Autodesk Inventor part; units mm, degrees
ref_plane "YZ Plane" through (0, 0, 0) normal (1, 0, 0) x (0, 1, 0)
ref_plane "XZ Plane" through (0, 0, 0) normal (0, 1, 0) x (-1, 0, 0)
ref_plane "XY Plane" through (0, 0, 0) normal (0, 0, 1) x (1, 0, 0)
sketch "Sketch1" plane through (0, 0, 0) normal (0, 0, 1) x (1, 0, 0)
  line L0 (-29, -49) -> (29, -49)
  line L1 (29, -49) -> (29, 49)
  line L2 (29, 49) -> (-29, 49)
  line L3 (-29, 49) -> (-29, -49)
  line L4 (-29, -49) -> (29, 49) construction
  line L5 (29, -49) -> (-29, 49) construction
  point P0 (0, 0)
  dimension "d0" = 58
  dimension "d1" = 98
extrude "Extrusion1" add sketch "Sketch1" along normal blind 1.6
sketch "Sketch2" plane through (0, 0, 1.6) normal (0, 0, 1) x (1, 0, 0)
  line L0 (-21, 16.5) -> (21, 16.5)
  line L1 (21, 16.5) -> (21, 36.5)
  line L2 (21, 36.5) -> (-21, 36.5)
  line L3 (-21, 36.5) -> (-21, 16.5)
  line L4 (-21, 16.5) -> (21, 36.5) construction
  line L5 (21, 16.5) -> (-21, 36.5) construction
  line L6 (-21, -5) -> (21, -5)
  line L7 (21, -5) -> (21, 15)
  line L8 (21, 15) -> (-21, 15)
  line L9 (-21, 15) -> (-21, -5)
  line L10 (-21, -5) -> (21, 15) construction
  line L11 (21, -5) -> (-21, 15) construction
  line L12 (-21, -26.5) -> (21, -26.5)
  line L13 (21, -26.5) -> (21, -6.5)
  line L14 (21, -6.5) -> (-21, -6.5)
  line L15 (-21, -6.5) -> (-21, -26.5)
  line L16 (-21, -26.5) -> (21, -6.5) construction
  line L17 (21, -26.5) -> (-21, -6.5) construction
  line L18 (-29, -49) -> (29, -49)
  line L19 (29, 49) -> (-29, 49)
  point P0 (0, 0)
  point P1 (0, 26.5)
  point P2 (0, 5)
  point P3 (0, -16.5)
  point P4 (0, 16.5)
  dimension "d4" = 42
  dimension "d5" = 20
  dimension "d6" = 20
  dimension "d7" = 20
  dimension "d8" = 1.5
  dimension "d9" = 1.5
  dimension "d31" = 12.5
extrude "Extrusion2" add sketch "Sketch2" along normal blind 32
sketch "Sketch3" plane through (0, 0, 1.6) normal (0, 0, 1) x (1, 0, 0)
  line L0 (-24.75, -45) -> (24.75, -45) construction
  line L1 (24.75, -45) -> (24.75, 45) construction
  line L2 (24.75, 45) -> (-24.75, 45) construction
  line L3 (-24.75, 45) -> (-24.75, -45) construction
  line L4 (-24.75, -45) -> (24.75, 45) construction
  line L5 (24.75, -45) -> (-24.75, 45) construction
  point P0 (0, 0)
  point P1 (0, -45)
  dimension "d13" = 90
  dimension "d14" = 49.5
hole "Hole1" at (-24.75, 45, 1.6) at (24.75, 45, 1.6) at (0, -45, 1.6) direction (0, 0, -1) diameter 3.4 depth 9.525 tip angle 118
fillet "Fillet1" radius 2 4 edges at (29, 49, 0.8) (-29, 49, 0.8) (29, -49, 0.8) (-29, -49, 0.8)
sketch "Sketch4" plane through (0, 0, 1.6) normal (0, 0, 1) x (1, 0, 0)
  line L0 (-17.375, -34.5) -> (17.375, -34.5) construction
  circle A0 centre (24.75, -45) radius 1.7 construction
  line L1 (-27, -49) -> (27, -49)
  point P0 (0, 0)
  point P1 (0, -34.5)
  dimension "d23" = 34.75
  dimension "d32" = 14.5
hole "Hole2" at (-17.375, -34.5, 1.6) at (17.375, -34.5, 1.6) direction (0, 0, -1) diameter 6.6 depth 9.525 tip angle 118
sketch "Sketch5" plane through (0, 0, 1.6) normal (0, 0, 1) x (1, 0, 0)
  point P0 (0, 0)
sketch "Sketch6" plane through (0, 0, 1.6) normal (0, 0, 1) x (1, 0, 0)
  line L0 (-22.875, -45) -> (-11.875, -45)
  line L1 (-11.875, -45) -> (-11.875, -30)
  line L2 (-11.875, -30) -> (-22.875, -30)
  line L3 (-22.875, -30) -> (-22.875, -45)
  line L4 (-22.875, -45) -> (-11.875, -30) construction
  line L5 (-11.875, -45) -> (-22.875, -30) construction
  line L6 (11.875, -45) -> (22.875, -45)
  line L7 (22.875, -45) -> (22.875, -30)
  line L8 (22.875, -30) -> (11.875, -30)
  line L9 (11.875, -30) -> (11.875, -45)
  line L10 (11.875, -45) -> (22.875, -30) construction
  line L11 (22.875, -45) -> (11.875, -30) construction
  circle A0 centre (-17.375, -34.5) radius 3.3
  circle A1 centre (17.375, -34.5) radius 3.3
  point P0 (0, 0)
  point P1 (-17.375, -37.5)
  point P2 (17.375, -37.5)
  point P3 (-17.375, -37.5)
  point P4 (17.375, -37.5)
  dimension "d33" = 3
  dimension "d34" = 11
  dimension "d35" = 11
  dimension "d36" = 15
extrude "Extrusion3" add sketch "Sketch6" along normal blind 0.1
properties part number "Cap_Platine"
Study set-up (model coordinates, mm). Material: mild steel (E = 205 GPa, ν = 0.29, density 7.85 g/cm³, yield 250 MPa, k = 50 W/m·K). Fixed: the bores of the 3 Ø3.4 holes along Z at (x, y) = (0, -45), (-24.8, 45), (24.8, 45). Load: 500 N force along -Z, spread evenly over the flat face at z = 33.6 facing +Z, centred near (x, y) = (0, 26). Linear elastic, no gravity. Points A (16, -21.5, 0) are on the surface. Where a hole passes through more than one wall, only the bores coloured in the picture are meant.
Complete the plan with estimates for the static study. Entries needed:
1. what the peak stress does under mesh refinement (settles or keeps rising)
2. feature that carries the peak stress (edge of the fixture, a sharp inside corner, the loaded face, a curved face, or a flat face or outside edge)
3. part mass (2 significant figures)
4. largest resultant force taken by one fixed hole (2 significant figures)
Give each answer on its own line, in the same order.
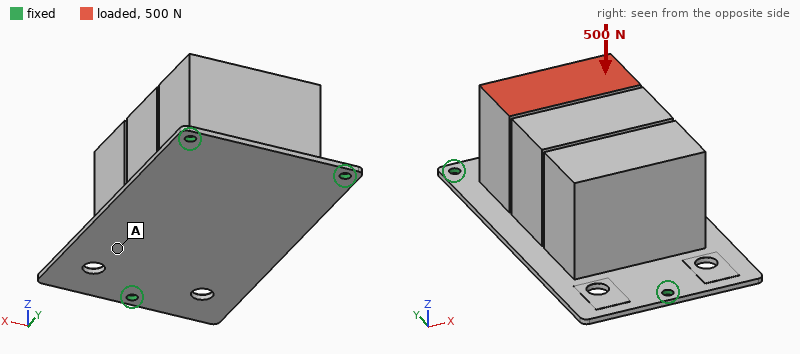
keeps rising
edge of the fixture
700 g
240 N
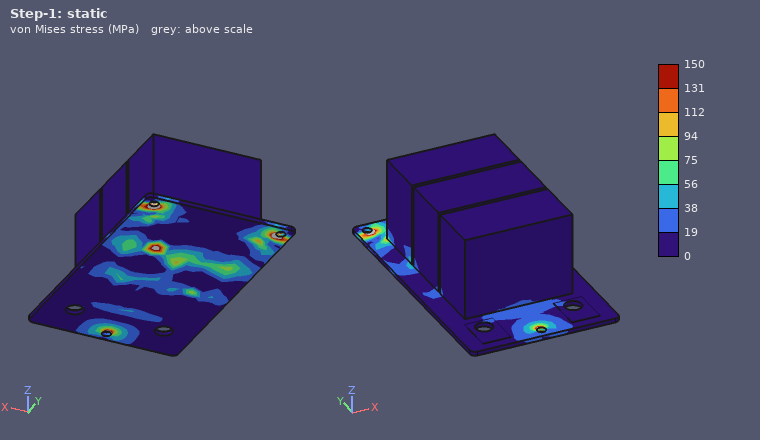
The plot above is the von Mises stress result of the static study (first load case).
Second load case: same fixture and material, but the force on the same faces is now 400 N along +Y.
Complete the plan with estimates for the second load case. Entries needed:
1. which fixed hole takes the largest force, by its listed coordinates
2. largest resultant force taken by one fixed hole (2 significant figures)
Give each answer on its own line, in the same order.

(0, -45)
420 N
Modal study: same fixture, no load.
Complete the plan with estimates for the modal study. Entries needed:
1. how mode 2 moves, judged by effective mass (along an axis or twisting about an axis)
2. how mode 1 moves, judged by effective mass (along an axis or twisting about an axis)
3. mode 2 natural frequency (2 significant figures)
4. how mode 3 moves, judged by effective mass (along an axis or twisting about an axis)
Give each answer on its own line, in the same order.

along X
along Z
820 Hz
along Y
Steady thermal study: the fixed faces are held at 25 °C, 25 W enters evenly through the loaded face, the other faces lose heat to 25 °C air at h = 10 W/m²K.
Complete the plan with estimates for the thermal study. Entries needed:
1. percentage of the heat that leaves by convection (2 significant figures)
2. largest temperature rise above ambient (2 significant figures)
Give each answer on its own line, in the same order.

39 %
77 K
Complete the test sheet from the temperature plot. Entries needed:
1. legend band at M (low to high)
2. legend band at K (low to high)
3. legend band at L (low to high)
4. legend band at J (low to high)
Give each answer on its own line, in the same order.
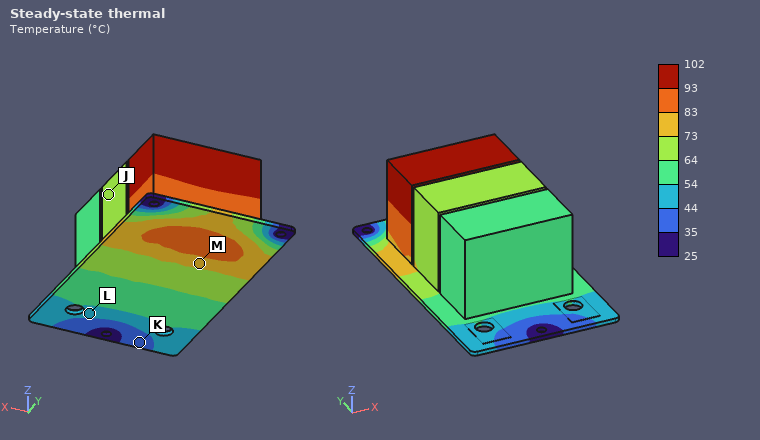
73 to 83 °C
35 to 44 °C
44 to 54 °C
64 to 73 °C
